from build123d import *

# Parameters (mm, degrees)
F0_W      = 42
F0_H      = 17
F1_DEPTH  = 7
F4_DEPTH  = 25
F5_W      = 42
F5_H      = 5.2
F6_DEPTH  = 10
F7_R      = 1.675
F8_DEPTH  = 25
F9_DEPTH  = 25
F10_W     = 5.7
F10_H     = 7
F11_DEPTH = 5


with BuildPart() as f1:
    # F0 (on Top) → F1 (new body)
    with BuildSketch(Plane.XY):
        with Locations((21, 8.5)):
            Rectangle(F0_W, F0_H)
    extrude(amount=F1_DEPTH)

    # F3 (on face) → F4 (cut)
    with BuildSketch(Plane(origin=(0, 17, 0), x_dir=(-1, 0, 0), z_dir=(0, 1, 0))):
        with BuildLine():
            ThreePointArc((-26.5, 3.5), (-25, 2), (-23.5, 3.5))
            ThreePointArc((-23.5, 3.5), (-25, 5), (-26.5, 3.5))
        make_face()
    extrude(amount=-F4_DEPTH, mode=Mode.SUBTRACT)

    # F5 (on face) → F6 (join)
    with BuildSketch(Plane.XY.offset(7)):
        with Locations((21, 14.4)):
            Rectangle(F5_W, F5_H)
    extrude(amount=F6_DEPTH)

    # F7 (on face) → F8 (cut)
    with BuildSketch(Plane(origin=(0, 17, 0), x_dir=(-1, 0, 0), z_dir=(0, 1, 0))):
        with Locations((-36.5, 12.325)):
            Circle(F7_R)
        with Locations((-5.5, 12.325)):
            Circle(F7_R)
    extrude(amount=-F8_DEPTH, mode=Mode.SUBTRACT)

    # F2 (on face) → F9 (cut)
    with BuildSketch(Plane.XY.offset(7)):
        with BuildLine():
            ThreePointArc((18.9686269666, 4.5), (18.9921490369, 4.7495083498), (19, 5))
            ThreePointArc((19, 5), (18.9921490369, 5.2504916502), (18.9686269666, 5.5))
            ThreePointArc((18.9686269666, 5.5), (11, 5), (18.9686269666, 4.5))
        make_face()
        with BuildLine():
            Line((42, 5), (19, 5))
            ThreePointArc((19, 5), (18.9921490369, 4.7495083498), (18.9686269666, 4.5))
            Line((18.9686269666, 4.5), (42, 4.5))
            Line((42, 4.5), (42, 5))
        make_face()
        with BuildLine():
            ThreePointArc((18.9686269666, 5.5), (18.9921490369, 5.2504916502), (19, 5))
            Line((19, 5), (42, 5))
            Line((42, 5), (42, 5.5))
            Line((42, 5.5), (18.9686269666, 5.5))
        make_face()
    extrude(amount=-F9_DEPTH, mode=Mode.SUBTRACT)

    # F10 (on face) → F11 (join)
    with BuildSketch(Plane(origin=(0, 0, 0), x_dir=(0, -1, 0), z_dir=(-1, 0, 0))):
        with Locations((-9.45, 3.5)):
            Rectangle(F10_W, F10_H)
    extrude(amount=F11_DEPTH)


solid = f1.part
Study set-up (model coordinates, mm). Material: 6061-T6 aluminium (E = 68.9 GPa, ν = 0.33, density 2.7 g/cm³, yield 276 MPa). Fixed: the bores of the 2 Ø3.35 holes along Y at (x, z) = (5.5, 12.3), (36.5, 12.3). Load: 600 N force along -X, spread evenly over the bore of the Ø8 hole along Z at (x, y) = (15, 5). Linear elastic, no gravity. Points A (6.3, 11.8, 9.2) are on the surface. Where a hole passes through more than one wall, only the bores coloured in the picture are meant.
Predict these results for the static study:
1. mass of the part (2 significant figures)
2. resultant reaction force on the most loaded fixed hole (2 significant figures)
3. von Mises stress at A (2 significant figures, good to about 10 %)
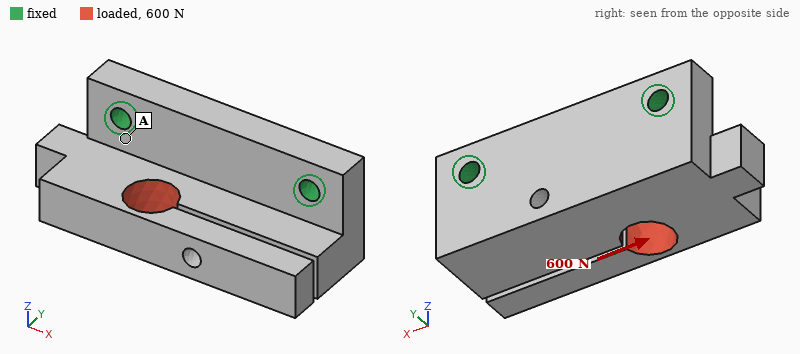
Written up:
18 g
370 N
23 MPa
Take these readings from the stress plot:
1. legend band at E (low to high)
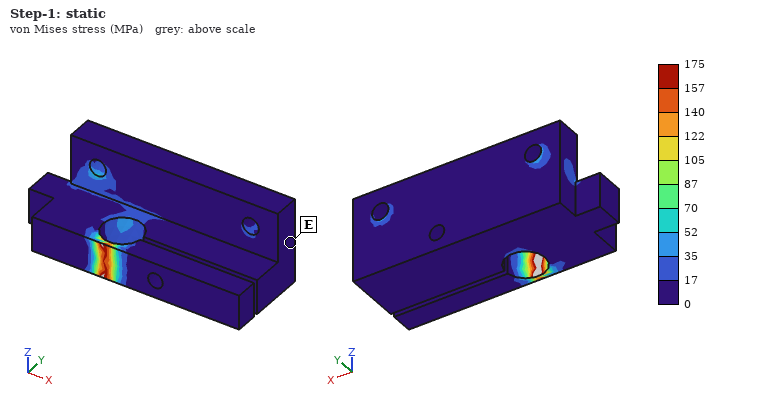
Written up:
0 to 17 MPa
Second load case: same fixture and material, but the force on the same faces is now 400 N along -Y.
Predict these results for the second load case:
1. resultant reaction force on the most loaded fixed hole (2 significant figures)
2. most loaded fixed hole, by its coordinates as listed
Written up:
290 N
(5.5, 12.3)
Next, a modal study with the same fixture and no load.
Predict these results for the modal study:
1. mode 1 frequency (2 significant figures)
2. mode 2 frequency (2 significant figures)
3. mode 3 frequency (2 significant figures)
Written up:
740 Hz
2600 Hz
7800 Hz
